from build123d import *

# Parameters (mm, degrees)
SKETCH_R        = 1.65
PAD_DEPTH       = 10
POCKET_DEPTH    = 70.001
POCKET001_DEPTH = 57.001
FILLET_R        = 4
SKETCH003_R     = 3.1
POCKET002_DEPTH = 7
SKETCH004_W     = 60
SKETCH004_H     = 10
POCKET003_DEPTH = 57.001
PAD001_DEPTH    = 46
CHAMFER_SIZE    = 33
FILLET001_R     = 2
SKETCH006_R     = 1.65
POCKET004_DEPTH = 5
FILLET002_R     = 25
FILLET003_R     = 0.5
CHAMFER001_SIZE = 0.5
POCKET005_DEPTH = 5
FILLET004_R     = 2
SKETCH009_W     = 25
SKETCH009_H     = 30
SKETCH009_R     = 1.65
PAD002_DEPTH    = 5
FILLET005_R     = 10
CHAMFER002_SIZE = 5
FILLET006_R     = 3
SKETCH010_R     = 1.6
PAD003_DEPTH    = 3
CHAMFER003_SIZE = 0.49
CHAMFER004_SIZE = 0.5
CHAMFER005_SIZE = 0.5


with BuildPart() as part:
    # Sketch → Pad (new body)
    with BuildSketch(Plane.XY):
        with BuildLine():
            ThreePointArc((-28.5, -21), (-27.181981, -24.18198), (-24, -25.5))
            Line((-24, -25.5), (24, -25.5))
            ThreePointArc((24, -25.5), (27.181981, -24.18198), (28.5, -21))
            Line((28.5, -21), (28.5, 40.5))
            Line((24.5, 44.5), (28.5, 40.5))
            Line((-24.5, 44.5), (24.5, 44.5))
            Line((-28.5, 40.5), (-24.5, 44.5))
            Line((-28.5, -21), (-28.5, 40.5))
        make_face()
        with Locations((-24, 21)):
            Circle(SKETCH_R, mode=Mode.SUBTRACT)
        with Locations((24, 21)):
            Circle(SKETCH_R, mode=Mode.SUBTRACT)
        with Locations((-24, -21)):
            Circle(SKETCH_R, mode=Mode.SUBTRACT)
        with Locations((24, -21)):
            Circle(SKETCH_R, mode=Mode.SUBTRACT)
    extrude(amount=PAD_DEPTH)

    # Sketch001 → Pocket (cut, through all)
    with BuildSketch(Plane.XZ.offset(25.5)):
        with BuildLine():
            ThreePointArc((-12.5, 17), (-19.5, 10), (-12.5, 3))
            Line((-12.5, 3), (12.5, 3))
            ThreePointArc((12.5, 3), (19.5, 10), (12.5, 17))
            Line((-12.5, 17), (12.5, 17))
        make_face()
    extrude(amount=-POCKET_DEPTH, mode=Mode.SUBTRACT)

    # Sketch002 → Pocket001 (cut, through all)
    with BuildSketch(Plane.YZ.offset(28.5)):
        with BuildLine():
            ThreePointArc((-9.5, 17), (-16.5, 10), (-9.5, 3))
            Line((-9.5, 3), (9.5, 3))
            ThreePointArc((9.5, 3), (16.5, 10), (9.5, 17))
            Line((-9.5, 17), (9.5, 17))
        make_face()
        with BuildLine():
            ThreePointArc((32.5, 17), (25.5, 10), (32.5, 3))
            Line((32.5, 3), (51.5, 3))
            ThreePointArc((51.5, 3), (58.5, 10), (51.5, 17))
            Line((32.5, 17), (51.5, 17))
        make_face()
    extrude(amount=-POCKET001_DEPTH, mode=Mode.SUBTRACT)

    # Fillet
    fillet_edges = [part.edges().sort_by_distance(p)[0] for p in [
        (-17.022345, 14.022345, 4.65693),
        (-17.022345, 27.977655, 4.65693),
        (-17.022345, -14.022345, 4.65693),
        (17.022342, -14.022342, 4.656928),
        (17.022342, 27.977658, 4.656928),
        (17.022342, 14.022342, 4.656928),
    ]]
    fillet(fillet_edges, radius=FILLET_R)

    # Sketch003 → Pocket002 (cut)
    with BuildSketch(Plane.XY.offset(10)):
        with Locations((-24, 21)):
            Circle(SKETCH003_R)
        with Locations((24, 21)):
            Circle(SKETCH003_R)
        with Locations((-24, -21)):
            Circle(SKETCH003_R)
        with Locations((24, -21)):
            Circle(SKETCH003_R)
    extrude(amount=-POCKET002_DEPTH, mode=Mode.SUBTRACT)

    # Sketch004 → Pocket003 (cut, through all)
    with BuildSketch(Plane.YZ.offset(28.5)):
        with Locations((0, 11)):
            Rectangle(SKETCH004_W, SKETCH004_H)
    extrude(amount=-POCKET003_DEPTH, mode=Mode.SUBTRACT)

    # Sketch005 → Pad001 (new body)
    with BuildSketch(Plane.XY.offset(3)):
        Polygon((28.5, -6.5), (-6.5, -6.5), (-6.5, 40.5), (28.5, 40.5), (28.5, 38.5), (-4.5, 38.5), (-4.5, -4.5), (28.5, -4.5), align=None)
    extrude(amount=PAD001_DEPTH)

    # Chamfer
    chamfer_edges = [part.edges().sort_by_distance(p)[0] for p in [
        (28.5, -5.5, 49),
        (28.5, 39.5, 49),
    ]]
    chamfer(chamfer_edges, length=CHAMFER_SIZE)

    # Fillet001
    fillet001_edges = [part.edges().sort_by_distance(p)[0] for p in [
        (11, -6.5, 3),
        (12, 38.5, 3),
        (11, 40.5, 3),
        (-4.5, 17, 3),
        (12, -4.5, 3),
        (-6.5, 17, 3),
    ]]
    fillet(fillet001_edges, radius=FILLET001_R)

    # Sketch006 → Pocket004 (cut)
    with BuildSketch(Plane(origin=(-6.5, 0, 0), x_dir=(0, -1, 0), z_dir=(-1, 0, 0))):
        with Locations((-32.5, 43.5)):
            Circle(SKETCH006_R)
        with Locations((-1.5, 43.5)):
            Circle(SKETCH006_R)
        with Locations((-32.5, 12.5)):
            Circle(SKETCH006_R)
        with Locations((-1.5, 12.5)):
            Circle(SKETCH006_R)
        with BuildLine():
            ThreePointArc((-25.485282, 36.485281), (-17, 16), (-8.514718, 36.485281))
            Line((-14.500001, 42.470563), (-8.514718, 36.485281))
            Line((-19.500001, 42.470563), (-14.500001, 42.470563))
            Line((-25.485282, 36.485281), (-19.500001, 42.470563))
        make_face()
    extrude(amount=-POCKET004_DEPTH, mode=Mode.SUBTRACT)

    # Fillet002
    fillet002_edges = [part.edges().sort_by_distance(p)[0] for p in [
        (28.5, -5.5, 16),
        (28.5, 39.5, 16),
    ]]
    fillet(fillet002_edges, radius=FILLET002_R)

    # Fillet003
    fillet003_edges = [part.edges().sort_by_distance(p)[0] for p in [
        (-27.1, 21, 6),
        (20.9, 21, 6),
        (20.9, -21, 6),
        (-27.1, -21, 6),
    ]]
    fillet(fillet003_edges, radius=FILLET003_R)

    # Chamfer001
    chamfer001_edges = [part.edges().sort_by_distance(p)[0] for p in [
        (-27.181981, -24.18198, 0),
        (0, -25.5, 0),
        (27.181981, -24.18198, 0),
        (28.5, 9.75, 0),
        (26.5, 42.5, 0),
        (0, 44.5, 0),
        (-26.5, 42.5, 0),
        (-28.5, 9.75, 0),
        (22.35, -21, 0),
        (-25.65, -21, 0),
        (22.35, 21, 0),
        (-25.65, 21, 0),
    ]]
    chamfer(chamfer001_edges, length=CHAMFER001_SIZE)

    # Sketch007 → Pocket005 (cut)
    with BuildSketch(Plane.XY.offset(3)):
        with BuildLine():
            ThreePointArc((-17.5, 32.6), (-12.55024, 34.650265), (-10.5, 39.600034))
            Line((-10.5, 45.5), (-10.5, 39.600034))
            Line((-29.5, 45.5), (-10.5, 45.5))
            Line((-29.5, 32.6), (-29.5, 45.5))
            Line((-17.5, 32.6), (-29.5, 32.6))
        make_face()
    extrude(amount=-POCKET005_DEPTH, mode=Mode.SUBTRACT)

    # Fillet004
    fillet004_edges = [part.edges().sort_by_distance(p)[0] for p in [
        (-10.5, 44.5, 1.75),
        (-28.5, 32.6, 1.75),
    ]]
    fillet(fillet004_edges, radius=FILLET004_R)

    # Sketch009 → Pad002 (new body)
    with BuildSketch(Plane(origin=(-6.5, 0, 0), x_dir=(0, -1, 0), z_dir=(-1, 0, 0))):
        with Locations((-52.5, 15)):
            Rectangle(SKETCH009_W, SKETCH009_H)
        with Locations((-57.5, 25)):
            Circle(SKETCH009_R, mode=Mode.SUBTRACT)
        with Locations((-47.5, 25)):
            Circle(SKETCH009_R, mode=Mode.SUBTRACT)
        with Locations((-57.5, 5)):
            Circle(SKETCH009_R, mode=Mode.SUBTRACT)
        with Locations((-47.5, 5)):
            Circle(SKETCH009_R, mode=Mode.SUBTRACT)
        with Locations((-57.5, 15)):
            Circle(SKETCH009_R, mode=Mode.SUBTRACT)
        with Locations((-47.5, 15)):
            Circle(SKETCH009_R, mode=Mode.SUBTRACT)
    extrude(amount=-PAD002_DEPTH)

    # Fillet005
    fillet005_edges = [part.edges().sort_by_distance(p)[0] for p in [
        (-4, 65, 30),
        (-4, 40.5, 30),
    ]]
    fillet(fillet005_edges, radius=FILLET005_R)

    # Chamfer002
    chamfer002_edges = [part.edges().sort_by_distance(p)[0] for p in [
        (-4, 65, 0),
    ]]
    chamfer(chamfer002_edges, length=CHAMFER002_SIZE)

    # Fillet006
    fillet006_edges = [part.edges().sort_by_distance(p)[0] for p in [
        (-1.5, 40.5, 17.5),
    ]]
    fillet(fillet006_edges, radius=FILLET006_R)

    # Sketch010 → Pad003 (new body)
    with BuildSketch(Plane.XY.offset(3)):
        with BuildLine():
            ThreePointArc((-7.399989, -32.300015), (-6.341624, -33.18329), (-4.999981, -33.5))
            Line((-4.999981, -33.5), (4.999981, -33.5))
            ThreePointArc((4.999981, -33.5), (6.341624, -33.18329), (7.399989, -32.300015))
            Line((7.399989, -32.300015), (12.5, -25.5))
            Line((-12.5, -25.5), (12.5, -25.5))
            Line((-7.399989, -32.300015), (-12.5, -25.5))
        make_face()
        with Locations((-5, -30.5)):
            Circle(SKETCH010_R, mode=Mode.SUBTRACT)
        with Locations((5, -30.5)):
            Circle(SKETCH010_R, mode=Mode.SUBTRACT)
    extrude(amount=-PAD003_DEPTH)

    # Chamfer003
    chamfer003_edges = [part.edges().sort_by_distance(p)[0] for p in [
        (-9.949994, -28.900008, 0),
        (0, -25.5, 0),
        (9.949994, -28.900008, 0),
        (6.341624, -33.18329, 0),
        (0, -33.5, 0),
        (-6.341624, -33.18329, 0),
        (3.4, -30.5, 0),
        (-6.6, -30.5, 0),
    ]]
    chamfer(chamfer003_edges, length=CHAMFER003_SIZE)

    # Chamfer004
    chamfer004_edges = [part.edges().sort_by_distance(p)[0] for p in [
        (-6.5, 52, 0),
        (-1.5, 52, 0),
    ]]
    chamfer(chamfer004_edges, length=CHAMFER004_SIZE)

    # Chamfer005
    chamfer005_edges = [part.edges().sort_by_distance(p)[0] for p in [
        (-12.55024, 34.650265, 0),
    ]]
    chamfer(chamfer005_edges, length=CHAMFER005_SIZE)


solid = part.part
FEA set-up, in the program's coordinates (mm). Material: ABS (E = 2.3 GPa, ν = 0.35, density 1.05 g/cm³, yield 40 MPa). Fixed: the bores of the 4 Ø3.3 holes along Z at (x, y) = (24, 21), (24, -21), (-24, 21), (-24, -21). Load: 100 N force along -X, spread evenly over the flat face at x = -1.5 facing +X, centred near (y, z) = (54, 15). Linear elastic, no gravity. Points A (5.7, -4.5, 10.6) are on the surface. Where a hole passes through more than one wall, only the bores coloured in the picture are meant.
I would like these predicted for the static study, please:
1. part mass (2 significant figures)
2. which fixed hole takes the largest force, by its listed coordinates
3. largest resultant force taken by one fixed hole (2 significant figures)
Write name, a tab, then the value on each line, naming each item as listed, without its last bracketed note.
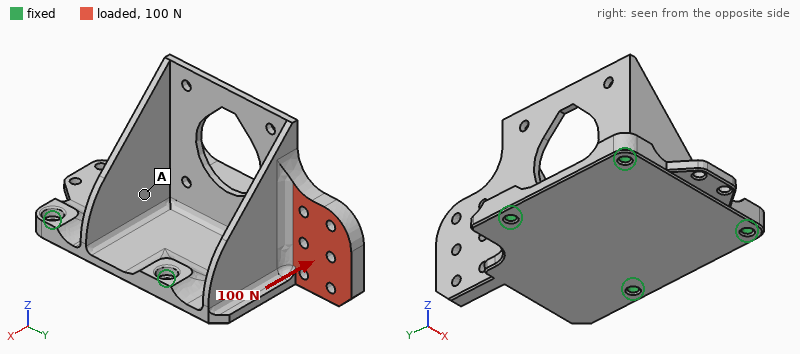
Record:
part mass	25 g
which fixed hole takes the largest force, by its listed coordinates	(24, 21)
largest resultant force taken by one fixed hole	100 N
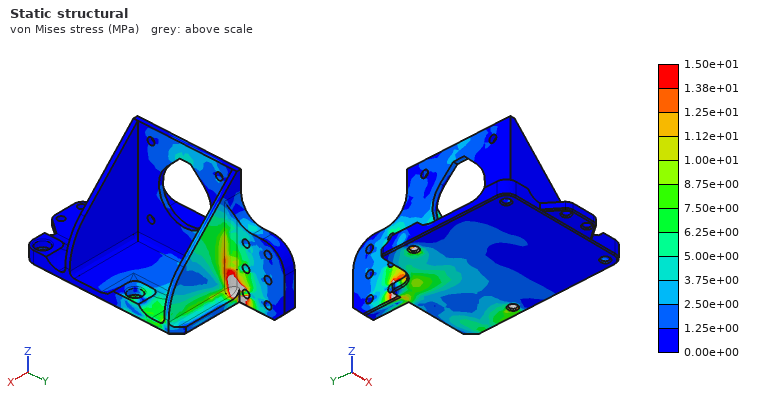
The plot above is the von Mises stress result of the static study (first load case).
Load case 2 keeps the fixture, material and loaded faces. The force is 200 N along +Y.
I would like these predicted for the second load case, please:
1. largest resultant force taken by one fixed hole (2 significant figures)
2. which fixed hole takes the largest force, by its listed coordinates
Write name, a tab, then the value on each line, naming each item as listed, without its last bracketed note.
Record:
largest resultant force taken by one fixed hole	81 N
which fixed hole takes the largest force, by its listed coordinates	(-24, 21)
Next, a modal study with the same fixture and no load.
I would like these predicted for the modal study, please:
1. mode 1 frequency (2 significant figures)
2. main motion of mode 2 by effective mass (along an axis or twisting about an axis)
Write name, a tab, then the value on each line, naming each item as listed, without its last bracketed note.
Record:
mode 1 frequency	510 Hz
main motion of mode 2 by effective mass	along X
